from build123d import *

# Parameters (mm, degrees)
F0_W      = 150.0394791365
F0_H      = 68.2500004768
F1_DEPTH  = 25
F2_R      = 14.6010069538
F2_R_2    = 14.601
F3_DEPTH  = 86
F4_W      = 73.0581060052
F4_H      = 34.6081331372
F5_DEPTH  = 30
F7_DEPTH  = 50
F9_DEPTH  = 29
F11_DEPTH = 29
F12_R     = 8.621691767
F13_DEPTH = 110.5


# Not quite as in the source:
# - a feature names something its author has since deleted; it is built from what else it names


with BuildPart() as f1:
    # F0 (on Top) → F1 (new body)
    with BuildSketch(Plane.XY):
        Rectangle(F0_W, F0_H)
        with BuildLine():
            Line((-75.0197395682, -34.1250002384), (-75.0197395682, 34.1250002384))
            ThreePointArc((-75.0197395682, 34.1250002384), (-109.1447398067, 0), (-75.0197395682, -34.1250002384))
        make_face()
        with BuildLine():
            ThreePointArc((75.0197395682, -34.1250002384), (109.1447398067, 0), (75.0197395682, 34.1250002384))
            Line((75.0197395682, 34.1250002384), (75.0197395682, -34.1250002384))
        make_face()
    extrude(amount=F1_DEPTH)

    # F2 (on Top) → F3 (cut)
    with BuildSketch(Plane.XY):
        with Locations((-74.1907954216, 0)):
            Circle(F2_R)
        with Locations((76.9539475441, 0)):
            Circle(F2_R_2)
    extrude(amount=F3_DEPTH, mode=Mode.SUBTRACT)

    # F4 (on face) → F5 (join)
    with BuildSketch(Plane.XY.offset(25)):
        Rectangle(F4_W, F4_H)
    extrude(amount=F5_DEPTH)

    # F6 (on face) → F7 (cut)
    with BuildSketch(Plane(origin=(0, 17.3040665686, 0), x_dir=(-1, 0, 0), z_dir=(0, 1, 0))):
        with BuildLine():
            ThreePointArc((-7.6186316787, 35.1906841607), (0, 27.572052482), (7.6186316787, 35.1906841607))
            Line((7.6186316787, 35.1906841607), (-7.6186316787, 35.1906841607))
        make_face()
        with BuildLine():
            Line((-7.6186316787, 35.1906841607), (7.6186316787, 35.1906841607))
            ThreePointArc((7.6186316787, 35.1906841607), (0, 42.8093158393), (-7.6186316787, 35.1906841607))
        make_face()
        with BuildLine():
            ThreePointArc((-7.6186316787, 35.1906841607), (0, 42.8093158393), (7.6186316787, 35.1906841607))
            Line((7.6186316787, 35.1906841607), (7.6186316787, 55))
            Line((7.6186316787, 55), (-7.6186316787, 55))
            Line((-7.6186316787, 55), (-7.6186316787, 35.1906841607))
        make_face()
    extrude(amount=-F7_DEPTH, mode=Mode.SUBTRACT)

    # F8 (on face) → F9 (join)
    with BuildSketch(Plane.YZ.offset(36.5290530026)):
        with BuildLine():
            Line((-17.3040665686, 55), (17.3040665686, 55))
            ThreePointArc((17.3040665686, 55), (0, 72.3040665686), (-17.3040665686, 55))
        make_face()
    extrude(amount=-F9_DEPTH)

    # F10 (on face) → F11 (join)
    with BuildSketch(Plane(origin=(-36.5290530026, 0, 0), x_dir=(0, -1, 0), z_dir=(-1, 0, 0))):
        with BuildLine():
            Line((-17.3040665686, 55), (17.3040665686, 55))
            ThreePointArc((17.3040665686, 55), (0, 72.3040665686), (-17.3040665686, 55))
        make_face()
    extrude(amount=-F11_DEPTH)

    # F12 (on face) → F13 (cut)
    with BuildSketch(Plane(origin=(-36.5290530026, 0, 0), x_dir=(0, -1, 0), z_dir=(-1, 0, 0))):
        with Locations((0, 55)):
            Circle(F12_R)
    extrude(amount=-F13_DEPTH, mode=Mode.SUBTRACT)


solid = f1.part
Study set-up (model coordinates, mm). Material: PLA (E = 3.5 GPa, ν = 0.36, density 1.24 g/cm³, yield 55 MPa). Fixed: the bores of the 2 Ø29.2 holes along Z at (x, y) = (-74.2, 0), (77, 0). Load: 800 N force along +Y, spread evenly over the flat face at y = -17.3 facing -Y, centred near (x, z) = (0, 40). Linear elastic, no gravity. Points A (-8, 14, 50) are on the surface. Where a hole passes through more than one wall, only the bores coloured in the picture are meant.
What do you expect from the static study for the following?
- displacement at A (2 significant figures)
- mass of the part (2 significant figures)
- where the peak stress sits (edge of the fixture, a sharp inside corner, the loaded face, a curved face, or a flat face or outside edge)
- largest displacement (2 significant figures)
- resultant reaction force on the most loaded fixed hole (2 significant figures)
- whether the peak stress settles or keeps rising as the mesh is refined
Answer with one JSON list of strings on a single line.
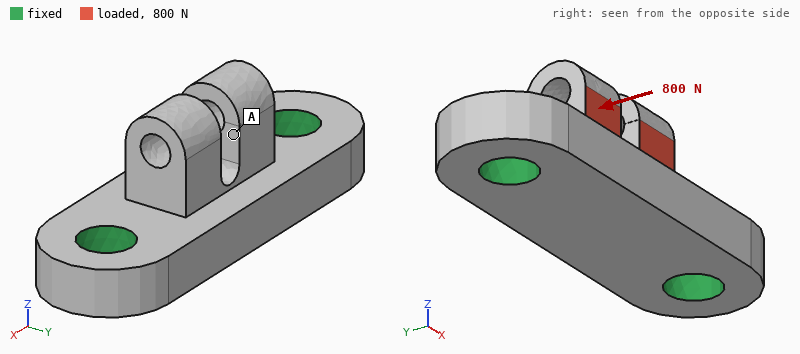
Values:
["59 µm", "480 g", "edge of the fixture", "88 µm", "410 N", "keeps rising"]
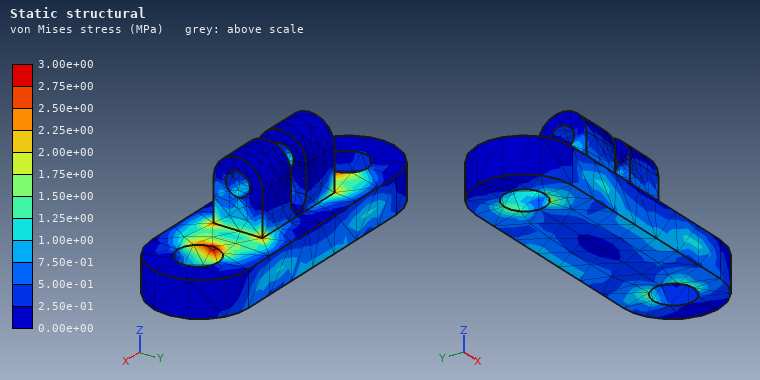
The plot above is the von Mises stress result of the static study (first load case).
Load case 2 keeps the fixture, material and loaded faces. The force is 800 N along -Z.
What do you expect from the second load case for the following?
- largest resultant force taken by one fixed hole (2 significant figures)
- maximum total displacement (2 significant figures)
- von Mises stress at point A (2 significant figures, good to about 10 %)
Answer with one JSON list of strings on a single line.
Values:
["420 N", "66 µm", "0.18 MPa"]
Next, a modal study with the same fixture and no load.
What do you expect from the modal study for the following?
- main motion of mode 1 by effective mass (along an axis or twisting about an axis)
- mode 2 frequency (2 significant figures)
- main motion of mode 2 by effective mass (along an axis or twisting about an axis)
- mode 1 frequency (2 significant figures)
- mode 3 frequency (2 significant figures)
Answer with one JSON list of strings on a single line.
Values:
["along Y", "1600 Hz", "along Z", "1500 Hz", "2600 Hz"]
